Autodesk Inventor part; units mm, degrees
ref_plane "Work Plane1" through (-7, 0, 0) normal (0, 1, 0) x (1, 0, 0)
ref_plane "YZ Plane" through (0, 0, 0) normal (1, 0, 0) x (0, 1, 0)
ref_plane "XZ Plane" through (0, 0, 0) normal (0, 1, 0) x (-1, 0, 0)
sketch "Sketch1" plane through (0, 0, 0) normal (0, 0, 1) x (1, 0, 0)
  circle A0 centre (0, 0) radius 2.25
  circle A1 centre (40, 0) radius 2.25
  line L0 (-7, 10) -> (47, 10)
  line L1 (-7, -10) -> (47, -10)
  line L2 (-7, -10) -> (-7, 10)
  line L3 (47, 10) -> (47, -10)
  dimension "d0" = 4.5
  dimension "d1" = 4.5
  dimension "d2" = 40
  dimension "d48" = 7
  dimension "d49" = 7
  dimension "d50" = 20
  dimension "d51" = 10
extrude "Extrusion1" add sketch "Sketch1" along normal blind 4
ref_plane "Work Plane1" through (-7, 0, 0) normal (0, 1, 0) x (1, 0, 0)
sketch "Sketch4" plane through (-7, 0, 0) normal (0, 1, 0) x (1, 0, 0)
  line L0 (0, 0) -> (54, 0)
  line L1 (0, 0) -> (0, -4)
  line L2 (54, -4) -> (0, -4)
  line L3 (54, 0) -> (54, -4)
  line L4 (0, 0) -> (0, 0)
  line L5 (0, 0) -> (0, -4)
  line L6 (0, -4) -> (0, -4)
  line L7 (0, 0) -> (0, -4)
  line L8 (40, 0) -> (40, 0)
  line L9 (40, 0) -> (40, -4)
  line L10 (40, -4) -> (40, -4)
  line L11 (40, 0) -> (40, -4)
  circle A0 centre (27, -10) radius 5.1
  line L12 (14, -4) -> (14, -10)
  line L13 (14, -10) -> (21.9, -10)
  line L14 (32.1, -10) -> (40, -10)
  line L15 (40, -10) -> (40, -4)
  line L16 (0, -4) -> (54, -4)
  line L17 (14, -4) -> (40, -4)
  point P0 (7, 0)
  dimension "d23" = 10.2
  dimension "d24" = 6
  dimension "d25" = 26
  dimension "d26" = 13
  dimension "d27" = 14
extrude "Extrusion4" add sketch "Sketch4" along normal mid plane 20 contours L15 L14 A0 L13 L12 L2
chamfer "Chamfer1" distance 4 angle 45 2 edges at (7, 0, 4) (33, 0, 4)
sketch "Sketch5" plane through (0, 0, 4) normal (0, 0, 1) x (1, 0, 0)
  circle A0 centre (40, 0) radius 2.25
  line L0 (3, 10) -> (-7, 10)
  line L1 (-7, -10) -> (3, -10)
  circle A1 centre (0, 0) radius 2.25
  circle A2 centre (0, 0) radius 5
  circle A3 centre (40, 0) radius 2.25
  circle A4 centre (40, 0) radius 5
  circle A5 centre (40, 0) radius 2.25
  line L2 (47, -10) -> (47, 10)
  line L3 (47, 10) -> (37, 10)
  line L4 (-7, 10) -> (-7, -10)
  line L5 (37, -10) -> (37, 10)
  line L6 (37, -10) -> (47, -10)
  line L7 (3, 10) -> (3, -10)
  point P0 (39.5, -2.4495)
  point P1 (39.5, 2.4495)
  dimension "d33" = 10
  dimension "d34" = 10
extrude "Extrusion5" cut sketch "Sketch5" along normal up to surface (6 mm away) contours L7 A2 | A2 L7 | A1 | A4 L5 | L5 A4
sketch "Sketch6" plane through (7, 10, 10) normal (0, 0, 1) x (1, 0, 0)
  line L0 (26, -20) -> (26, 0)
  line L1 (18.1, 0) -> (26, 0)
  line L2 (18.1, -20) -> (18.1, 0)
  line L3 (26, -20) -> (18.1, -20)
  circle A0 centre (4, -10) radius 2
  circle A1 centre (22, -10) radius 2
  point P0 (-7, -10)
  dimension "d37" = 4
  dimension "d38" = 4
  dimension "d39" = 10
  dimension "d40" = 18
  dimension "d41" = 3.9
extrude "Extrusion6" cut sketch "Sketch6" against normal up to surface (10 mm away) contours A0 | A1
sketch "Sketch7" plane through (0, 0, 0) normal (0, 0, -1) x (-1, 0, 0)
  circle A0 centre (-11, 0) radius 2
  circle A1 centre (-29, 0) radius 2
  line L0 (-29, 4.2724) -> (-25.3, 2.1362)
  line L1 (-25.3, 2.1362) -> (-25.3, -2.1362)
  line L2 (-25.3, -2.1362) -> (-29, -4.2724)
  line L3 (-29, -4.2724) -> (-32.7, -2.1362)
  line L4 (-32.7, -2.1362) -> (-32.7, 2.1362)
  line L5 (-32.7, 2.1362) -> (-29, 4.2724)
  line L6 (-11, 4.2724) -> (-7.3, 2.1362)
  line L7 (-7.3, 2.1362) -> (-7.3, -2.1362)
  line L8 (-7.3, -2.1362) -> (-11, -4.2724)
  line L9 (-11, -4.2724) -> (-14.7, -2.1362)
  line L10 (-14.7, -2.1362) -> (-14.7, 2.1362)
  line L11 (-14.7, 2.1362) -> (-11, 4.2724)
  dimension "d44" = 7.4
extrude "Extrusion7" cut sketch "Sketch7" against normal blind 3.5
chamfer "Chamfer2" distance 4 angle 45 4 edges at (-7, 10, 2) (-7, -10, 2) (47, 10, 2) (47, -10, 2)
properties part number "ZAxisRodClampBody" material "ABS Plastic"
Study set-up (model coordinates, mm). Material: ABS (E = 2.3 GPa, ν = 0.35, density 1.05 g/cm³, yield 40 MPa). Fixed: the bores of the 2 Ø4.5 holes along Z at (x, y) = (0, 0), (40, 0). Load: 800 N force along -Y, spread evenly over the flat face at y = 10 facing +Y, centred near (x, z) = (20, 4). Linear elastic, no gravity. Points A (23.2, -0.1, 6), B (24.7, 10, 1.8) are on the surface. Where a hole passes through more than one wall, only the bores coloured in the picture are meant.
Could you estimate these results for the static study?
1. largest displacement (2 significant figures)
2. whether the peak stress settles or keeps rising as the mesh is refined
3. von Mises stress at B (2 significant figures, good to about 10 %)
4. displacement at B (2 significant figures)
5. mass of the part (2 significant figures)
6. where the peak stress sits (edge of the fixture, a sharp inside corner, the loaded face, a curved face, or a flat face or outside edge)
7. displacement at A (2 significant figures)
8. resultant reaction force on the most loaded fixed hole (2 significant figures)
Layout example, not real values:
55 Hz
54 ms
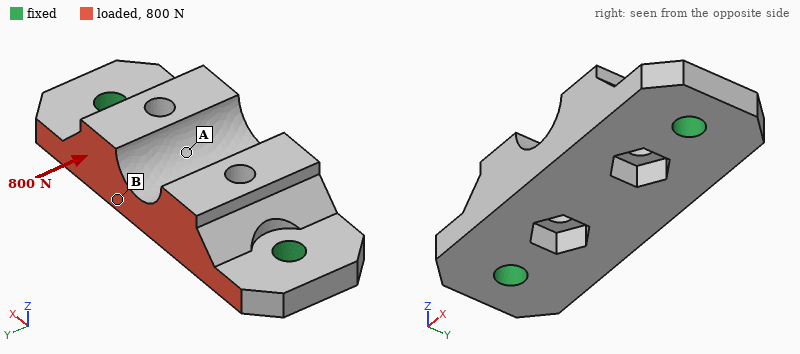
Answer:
0.20 mm
keeps rising
8.9 MPa
0.13 mm
6.5 g
edge of the fixture
0.13 mm
400 N
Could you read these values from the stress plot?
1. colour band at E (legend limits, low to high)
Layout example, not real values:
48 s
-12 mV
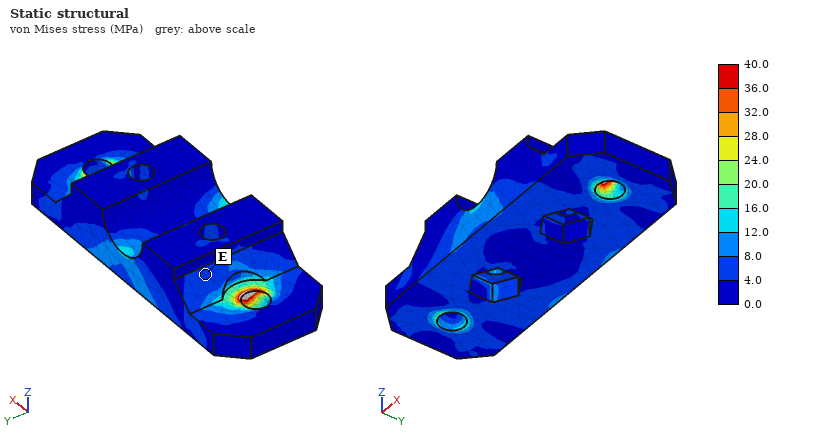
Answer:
4.0 to 8.0 MPa
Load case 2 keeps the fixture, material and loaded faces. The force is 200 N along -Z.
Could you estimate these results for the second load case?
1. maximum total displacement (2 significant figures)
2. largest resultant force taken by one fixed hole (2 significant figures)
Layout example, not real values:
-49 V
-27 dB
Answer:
0.26 mm
120 N
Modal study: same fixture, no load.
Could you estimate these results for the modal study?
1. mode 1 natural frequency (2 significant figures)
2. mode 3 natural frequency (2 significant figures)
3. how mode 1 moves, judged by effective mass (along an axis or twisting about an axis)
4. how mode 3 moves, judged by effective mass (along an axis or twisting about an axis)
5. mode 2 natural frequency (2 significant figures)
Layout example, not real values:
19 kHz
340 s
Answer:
3500 Hz
6100 Hz
along Z
along Y
3700 Hz
